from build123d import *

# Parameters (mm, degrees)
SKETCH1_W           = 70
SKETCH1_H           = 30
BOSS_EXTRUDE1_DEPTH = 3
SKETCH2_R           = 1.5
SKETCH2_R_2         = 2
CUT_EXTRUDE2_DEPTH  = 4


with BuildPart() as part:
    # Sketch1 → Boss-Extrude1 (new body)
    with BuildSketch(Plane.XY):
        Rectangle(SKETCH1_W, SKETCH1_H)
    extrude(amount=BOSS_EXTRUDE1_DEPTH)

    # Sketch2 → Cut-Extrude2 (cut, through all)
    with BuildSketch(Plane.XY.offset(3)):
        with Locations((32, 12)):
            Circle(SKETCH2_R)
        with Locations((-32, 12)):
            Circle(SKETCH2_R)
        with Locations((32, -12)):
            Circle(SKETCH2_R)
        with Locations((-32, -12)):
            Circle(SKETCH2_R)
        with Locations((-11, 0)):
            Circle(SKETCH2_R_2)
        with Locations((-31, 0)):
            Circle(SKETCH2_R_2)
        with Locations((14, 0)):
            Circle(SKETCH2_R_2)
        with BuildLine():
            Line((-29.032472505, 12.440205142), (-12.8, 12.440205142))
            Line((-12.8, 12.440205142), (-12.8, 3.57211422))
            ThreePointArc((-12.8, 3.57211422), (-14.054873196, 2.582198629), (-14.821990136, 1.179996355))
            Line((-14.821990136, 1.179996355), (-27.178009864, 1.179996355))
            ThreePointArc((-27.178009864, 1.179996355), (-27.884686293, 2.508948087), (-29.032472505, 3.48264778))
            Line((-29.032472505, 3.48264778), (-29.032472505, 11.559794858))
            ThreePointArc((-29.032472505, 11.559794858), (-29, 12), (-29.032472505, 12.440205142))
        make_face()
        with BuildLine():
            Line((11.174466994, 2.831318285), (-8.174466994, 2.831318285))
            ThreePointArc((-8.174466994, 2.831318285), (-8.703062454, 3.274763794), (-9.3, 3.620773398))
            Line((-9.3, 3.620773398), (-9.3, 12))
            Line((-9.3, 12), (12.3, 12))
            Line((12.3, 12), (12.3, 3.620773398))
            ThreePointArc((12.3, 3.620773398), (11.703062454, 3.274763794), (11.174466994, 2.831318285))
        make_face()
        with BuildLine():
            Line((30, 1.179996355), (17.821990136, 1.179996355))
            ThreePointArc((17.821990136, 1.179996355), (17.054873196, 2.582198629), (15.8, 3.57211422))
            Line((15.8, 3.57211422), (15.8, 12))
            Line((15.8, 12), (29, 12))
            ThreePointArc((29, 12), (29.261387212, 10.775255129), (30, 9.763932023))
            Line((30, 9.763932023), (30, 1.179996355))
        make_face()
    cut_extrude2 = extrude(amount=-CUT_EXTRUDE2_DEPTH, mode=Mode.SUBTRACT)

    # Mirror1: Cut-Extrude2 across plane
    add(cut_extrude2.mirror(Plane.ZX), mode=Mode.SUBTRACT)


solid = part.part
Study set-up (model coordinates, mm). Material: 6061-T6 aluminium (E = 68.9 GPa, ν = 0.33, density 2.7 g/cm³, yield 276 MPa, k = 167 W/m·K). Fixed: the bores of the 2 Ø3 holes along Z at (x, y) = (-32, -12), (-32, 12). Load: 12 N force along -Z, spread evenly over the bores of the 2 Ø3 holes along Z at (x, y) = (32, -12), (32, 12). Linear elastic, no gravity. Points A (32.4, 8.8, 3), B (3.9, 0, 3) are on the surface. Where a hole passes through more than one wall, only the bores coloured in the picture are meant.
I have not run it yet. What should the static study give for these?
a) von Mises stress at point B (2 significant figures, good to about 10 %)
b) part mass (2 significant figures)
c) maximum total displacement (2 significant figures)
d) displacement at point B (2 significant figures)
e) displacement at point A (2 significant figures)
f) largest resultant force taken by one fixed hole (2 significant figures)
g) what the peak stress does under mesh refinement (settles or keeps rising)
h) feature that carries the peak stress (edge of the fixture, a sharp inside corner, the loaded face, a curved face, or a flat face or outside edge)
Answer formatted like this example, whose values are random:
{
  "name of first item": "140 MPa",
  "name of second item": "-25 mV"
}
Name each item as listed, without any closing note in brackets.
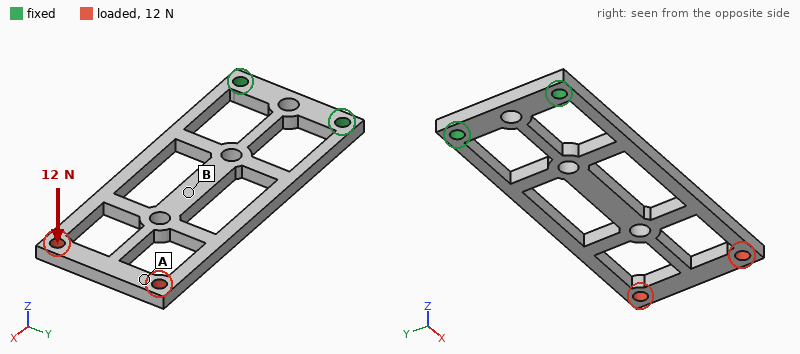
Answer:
{
  "von Mises stress at point B": "16 MPa",
  "part mass": "8.0 g",
  "maximum total displacement": "0.85 mm",
  "displacement at point B": "0.32 mm",
  "displacement at point A": "0.80 mm",
  "largest resultant force taken by one fixed hole": "6.0 N",
  "what the peak stress does under mesh refinement": "keeps rising",
  "feature that carries the peak stress": "a sharp inside corner"
}
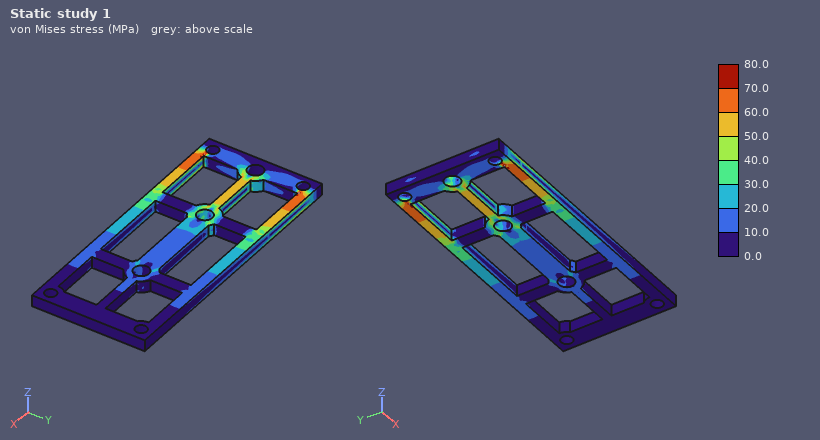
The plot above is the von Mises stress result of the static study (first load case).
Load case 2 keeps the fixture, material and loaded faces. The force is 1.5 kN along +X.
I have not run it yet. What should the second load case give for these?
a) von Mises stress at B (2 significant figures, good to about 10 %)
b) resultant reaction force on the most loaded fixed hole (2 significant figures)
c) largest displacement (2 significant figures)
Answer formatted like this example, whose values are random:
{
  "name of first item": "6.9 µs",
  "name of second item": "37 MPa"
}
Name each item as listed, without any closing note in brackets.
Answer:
{
  "von Mises stress at B": "22 MPa",
  "resultant reaction force on the most loaded fixed hole": "750 N",
  "largest displacement": "67 µm"
}
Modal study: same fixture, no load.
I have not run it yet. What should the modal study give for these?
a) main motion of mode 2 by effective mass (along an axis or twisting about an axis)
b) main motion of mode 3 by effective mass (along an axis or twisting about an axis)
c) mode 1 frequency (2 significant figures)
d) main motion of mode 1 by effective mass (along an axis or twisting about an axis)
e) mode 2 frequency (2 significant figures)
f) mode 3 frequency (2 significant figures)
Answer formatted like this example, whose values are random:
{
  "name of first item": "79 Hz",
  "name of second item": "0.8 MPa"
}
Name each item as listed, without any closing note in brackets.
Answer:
{
  "main motion of mode 2 by effective mass": "twisting about X",
  "main motion of mode 3 by effective mass": "along Y",
  "mode 1 frequency": "400 Hz",
  "main motion of mode 1 by effective mass": "along Z",
  "mode 2 frequency": "1700 Hz",
  "mode 3 frequency": "1900 Hz"
}
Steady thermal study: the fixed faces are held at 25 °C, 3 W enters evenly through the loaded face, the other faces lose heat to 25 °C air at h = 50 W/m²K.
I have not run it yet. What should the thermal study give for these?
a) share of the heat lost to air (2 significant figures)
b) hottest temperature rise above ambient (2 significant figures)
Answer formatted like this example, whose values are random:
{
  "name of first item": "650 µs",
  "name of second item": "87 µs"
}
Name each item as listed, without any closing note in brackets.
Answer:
{
  "share of the heat lost to air": "61 %",
  "hottest temperature rise above ambient": "23 K"
}
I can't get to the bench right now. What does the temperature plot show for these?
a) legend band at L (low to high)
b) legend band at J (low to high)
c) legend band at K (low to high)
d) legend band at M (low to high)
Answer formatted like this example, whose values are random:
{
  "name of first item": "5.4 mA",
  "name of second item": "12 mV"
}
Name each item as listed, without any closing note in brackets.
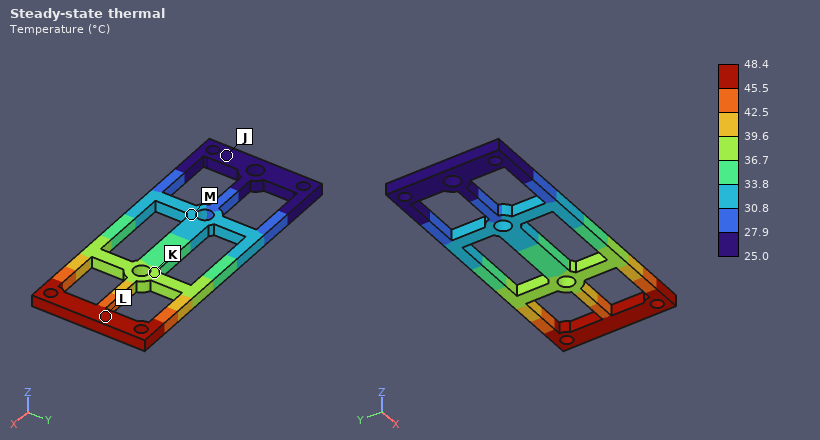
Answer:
{
  "legend band at L": "45.5 to 48.4 °C",
  "legend band at J": "25.0 to 27.9 °C",
  "legend band at K": "36.7 to 39.6 °C",
  "legend band at M": "30.8 to 33.8 °C"
}
